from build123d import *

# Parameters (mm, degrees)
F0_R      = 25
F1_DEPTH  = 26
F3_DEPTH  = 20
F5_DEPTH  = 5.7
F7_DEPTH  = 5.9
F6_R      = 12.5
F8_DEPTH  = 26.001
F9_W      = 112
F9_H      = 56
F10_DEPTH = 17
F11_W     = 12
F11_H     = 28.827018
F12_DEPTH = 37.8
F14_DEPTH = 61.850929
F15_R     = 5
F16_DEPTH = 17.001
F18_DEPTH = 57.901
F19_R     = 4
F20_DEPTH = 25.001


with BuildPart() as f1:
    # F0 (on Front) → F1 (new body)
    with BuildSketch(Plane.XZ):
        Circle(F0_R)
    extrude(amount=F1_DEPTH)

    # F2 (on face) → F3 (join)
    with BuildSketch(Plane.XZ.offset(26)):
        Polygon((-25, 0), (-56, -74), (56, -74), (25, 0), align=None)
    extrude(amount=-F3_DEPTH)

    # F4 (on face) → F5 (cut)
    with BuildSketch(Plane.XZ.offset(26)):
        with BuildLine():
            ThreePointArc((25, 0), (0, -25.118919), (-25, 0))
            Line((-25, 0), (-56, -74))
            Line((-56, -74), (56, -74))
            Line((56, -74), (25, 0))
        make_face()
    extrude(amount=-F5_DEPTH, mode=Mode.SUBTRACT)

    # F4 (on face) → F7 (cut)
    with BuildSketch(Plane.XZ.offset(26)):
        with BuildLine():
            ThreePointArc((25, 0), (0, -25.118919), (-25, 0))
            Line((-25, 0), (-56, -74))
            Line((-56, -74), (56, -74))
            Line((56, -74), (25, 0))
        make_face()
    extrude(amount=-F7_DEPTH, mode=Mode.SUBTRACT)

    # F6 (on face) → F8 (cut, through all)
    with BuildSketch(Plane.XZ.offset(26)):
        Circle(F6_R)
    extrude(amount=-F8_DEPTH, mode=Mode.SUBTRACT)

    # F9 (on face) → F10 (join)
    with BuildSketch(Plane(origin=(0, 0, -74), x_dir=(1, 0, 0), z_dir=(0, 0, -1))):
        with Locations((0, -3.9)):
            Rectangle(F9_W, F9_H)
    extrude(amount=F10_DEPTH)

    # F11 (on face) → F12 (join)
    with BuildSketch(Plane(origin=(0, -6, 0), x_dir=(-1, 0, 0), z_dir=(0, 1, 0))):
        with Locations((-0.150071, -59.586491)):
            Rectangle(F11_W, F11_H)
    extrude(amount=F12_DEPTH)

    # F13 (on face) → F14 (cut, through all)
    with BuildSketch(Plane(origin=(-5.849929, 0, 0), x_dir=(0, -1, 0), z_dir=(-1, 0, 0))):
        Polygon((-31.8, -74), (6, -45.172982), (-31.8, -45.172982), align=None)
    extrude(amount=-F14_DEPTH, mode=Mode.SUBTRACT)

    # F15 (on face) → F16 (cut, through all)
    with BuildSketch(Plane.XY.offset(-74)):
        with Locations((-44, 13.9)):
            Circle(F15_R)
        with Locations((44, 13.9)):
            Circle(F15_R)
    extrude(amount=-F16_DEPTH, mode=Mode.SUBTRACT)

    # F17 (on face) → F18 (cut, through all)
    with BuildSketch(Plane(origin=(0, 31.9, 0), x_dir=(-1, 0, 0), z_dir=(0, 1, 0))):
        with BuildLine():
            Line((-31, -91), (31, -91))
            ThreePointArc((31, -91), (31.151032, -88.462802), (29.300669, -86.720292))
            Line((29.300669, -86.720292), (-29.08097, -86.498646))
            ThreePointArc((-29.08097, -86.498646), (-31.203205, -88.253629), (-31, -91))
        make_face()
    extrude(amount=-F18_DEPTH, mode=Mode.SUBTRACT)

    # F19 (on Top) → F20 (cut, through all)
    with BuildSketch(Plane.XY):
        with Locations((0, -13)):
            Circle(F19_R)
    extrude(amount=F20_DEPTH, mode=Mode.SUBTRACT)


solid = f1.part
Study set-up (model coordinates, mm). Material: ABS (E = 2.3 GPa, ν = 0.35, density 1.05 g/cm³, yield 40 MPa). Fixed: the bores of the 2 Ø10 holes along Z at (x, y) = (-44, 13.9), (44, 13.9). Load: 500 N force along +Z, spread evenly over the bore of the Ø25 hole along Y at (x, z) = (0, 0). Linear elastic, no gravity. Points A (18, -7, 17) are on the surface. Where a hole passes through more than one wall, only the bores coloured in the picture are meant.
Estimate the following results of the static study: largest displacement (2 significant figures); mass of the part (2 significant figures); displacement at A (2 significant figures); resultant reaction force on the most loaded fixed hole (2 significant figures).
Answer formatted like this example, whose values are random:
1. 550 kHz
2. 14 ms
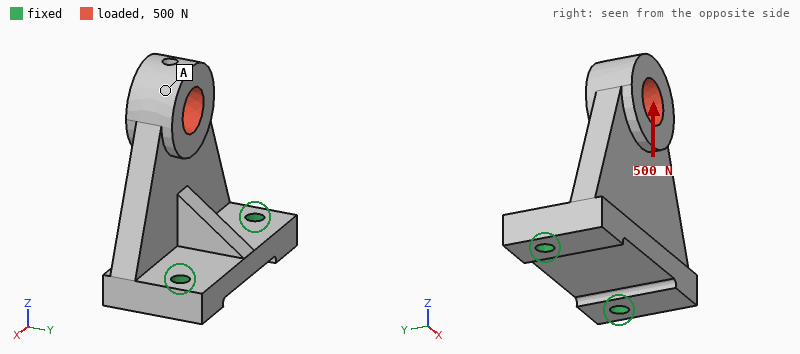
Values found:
1. 0.30 mm
2. 210 g
3. 0.26 mm
4. 250 N
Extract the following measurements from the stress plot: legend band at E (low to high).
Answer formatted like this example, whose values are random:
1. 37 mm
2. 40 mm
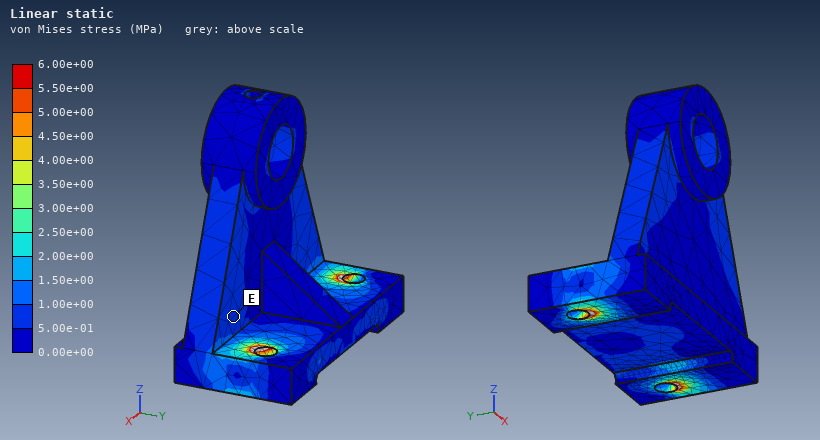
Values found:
1. 5.00e-01 to 1.00e+00 MPa
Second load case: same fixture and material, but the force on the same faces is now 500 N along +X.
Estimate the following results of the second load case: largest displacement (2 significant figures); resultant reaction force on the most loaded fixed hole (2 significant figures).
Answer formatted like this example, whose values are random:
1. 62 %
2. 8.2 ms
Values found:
1. 0.30 mm
2. 550 N
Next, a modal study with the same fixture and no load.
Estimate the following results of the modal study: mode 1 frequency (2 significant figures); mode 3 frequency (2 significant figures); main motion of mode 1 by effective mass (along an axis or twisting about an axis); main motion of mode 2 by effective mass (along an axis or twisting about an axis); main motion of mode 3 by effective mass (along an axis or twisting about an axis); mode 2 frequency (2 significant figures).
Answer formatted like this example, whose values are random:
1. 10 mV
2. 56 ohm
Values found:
1. 340 Hz
2. 1200 Hz
3. along Y
4. along X
5. along Z
6. 940 Hz
